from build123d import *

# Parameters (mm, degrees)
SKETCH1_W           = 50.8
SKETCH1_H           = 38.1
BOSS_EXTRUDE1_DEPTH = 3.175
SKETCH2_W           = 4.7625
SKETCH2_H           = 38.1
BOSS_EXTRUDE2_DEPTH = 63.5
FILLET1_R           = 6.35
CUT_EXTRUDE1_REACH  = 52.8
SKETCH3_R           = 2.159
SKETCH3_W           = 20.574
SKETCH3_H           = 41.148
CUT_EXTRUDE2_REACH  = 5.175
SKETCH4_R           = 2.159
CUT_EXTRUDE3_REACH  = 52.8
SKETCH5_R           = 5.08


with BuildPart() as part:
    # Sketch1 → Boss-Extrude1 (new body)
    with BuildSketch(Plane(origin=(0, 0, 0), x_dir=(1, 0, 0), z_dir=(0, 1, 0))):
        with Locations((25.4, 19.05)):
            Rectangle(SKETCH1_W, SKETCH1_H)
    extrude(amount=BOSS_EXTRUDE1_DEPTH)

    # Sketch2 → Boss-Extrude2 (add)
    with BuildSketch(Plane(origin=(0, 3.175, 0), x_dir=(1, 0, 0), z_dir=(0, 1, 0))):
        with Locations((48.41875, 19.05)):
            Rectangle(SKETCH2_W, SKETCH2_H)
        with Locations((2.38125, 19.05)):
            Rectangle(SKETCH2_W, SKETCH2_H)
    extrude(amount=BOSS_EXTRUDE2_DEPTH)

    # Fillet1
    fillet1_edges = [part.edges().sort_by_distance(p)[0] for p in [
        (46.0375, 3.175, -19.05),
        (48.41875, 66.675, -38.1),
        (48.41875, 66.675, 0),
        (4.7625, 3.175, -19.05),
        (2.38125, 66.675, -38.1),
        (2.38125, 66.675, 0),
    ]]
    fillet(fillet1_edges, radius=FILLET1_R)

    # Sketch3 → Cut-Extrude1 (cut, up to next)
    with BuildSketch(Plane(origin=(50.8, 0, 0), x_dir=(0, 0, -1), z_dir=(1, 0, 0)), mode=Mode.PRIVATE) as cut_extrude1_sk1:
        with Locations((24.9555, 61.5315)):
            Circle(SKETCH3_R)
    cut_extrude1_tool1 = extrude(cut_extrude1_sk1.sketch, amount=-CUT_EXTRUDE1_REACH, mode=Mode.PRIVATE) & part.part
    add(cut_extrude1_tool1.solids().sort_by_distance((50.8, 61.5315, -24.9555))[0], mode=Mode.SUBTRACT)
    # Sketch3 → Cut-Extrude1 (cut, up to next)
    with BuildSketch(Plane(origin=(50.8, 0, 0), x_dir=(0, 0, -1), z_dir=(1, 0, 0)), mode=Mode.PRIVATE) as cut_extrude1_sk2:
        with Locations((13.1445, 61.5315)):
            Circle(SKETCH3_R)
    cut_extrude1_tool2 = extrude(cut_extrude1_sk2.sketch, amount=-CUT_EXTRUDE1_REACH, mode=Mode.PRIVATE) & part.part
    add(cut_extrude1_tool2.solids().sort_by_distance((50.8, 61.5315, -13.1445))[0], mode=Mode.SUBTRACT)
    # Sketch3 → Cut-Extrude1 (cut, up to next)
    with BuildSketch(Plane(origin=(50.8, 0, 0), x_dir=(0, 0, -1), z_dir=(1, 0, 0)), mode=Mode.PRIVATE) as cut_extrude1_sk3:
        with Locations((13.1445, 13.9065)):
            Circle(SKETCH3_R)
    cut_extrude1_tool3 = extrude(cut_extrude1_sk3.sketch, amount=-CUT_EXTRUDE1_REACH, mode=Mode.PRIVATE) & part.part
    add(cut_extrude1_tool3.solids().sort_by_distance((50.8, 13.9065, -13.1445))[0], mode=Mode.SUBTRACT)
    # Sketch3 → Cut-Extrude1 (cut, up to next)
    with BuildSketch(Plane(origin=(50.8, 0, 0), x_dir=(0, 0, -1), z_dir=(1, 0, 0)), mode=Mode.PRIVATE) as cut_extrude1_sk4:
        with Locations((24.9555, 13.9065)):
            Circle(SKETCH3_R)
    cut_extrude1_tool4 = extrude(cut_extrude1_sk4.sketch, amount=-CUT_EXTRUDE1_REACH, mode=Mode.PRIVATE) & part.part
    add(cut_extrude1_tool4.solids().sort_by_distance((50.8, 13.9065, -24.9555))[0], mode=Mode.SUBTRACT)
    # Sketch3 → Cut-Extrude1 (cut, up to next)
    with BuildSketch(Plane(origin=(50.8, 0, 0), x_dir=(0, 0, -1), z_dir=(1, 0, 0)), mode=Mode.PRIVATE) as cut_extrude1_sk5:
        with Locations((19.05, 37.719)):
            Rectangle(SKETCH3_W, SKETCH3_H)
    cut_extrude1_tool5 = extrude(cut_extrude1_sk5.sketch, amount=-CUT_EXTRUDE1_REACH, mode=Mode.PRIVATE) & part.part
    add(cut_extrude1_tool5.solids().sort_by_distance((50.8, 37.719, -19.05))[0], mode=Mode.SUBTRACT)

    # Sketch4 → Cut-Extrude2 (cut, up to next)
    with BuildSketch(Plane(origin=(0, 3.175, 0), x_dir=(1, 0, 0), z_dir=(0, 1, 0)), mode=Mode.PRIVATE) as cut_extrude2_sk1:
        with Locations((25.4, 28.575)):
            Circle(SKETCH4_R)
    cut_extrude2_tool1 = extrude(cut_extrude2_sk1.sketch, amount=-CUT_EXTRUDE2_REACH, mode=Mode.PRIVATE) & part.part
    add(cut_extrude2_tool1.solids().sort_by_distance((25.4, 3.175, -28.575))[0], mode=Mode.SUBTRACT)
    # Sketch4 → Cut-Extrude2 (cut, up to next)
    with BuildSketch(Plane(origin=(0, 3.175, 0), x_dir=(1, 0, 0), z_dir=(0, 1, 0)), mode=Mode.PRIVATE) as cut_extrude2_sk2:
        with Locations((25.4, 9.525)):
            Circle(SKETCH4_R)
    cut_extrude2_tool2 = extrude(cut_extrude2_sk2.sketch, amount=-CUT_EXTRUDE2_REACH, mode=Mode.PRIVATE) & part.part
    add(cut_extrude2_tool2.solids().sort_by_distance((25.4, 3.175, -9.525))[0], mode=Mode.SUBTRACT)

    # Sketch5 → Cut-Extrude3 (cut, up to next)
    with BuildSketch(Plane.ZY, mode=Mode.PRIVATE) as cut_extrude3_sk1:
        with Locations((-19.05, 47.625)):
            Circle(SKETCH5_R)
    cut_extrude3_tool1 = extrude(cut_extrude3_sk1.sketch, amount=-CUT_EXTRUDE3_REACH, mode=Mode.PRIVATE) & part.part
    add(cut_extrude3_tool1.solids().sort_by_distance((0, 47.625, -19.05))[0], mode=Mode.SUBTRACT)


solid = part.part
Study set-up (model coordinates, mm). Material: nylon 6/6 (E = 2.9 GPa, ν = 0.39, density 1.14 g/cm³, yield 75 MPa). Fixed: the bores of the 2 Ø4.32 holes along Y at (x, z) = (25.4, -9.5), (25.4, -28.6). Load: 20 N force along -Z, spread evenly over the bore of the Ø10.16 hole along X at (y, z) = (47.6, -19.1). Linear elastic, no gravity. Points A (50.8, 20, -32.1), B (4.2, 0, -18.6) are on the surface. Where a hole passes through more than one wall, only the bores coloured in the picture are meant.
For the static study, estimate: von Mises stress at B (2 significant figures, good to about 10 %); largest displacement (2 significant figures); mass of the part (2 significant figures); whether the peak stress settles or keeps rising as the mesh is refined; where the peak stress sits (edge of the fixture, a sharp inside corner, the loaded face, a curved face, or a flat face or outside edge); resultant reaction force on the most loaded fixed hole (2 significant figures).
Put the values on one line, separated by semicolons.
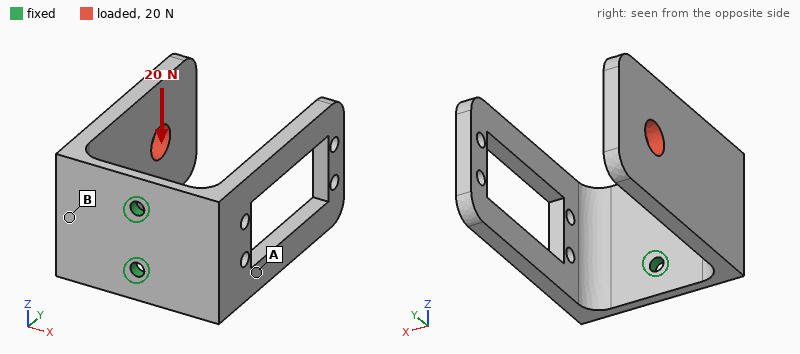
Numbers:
3.6 MPa; 0.96 mm; 28 g; keeps rising; edge of the fixture; 44 N
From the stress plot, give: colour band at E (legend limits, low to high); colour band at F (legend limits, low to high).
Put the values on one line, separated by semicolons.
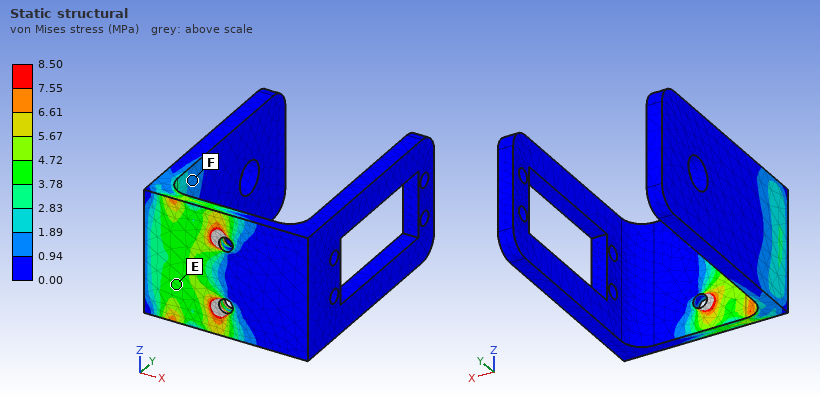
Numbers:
3.78 to 4.72 MPa; 0.94 to 1.89 MPa
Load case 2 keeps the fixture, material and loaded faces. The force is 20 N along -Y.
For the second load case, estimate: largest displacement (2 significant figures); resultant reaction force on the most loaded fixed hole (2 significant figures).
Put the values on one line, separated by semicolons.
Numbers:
1.0 mm; 10 N
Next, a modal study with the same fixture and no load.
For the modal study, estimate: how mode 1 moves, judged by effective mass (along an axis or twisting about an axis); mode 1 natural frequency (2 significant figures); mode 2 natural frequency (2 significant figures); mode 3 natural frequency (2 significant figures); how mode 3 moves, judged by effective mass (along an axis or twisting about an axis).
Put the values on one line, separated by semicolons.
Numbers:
along X; 140 Hz; 160 Hz; 290 Hz; along Z
